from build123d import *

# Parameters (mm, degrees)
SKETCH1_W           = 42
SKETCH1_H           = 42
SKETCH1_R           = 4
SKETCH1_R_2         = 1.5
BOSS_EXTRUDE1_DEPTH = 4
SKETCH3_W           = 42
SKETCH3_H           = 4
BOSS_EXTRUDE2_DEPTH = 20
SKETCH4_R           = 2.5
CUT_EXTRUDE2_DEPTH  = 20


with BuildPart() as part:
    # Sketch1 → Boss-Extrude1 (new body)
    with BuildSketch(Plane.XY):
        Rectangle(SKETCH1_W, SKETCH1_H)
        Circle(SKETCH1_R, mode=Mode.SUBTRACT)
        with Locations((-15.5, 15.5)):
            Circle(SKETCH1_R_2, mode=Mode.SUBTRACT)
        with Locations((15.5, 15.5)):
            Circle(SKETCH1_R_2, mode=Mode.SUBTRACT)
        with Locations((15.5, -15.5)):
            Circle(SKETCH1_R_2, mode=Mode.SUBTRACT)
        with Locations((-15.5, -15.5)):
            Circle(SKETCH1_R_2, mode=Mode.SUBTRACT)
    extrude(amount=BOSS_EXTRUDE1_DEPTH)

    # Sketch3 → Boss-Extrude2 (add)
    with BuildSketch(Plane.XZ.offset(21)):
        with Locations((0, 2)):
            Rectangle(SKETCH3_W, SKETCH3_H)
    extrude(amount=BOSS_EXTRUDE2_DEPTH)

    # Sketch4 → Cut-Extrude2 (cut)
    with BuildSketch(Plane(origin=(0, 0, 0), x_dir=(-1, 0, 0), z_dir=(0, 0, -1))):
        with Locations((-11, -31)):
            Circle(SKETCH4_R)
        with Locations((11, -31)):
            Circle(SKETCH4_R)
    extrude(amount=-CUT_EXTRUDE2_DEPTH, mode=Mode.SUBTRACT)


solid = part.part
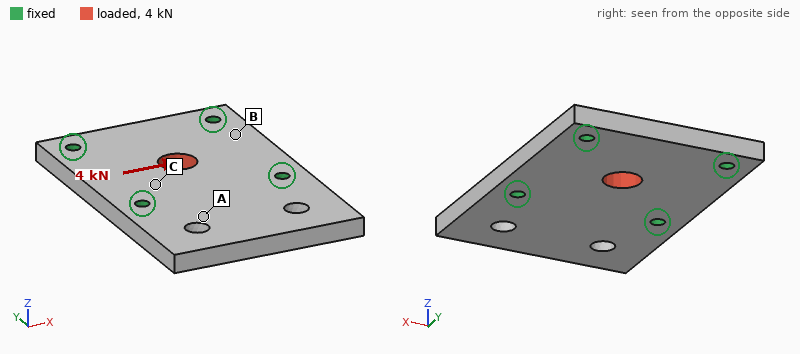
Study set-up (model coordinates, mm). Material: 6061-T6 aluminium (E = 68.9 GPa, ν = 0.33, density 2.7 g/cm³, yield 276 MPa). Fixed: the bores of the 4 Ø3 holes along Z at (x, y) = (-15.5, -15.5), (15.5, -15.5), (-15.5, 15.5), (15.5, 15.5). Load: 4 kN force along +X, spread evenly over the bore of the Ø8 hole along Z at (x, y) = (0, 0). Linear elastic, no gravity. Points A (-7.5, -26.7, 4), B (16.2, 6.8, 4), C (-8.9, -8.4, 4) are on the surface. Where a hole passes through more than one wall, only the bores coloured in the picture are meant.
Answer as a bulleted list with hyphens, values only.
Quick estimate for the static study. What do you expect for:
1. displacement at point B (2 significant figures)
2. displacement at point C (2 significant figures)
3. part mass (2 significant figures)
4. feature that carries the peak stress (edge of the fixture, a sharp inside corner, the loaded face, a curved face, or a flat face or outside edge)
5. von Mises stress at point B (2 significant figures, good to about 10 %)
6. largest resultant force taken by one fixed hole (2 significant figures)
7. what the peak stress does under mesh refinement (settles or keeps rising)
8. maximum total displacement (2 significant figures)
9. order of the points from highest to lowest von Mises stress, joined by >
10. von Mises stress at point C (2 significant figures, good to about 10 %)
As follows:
- 5.2 µm
- 4.9 µm
- 27 g
- edge of the fixture
- 14 MPa
- 1.1 kN
- keeps rising
- 10 µm
- C > B > A
- 28 MPa
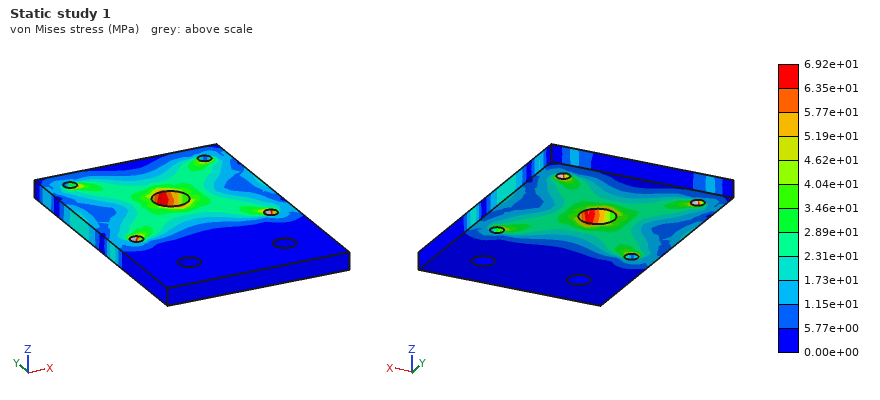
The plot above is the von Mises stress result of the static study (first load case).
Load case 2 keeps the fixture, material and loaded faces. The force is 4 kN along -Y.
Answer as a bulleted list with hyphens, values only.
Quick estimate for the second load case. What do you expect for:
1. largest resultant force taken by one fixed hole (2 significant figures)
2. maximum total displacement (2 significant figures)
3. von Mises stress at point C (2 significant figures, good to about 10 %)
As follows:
- 1.1 kN
- 10 µm
- 24 MPa
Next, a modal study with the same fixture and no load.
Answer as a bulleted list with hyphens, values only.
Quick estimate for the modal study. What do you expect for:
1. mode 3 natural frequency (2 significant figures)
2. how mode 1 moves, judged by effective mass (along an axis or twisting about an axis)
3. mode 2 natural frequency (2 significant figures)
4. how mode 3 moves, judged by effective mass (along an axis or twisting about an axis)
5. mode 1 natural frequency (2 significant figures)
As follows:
- 14 kHz
- along Z
- 8200 Hz
- along Z
- 4500 Hz
